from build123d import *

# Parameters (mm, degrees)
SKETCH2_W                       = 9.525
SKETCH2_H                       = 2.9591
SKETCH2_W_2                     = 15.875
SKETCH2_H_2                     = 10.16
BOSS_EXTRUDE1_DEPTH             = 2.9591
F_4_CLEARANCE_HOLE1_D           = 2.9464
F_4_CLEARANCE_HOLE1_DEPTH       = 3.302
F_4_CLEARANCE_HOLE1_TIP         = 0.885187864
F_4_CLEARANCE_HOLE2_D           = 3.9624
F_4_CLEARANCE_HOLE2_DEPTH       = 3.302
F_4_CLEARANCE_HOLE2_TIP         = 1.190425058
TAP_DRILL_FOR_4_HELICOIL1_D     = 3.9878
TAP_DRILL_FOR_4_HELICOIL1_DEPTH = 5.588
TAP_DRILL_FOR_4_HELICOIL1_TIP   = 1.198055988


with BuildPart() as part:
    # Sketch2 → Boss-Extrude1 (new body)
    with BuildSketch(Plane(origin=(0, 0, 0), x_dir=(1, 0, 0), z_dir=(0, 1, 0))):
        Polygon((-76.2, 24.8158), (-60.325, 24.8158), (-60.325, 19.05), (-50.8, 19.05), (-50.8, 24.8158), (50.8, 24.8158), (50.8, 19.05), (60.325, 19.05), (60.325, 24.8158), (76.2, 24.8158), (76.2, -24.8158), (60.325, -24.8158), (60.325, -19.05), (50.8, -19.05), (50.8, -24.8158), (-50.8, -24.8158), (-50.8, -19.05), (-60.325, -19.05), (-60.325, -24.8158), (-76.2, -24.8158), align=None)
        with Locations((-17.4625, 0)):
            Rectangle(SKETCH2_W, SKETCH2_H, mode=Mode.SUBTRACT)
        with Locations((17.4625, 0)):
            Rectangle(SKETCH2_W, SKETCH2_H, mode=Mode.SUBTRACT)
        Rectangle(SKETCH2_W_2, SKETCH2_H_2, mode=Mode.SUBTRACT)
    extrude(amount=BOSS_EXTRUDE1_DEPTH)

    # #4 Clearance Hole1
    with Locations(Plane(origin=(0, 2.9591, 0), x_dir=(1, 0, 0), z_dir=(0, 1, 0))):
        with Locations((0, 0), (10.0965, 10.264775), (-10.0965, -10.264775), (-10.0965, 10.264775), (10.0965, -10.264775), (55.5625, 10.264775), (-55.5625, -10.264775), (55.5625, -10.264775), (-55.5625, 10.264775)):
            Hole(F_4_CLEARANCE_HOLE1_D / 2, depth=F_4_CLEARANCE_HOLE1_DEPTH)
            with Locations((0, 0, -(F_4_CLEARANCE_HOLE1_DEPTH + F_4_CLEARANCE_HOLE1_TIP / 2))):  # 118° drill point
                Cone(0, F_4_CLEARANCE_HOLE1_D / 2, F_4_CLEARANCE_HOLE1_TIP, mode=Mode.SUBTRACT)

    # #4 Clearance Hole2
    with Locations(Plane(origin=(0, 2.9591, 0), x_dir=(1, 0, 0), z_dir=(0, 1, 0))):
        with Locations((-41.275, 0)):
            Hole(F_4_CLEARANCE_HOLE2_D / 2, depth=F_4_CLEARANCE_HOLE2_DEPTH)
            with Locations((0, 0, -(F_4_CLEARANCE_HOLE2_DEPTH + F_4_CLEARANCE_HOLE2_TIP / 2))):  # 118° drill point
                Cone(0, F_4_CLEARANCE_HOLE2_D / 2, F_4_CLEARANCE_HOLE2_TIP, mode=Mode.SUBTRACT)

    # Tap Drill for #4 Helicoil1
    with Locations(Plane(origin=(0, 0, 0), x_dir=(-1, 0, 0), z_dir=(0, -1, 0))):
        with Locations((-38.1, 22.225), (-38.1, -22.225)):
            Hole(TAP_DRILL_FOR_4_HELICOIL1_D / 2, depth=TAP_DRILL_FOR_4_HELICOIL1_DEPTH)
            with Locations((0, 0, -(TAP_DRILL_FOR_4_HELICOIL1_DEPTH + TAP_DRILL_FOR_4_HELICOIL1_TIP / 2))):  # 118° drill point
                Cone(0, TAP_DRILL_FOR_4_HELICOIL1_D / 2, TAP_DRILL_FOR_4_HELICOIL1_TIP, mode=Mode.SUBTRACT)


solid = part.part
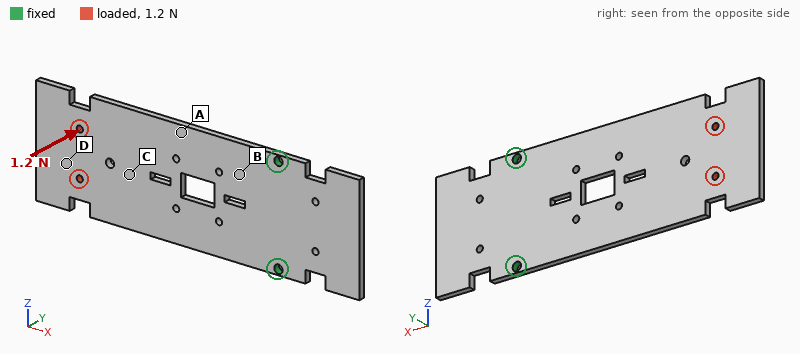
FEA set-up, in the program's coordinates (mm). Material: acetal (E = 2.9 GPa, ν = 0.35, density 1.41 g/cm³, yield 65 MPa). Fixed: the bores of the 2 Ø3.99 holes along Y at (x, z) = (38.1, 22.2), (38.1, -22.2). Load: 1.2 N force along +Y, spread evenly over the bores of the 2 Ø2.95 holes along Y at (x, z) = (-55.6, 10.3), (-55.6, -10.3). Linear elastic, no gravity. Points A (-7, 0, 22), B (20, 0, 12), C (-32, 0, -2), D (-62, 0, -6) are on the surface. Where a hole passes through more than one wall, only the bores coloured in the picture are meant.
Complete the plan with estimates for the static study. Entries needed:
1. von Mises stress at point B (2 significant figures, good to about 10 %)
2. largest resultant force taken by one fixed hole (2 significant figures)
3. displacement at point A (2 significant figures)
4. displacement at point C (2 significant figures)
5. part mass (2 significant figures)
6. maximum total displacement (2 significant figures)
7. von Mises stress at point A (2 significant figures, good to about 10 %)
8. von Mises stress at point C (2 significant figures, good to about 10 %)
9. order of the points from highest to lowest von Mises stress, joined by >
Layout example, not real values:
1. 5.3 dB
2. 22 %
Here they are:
1. 1.2 MPa
2. 0.60 N
3. 0.38 mm
4. 0.82 mm
5. 29 g
6. 1.7 mm
7. 1.0 MPa
8. 0.40 MPa
9. B > A > C > D
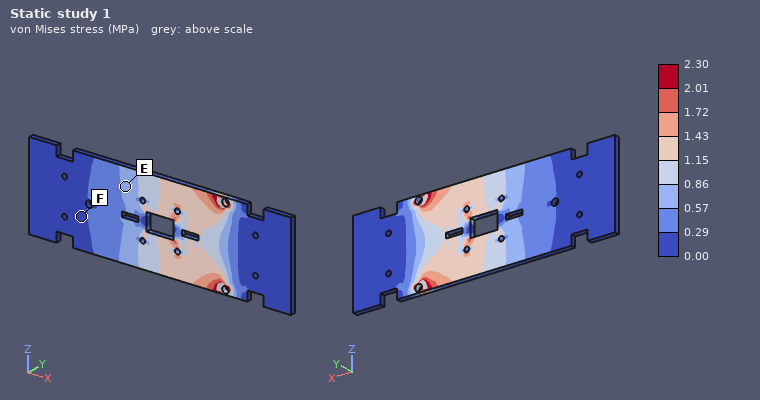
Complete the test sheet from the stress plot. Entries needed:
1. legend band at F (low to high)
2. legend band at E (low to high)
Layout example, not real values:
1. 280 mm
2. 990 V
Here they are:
1. 0.00 to 0.29 MPa
2. 0.57 to 0.86 MPa
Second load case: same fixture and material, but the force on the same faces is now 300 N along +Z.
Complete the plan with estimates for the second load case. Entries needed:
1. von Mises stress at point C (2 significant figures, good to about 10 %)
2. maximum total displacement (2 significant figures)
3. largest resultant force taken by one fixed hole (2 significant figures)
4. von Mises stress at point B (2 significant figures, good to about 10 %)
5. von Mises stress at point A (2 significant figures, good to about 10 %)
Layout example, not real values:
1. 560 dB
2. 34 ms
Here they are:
1. 7.4 MPa
2. 1.7 mm
3. 650 N
4. 7.6 MPa
5. 9.4 MPa
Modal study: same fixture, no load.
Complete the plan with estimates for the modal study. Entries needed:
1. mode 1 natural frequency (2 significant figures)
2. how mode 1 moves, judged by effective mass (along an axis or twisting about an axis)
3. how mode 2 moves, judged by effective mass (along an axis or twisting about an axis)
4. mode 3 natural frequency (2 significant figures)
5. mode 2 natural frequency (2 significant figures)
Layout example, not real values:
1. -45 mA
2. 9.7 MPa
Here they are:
1. 49 Hz
2. along Y
3. twisting about X
4. 310 Hz
5. 250 Hz
